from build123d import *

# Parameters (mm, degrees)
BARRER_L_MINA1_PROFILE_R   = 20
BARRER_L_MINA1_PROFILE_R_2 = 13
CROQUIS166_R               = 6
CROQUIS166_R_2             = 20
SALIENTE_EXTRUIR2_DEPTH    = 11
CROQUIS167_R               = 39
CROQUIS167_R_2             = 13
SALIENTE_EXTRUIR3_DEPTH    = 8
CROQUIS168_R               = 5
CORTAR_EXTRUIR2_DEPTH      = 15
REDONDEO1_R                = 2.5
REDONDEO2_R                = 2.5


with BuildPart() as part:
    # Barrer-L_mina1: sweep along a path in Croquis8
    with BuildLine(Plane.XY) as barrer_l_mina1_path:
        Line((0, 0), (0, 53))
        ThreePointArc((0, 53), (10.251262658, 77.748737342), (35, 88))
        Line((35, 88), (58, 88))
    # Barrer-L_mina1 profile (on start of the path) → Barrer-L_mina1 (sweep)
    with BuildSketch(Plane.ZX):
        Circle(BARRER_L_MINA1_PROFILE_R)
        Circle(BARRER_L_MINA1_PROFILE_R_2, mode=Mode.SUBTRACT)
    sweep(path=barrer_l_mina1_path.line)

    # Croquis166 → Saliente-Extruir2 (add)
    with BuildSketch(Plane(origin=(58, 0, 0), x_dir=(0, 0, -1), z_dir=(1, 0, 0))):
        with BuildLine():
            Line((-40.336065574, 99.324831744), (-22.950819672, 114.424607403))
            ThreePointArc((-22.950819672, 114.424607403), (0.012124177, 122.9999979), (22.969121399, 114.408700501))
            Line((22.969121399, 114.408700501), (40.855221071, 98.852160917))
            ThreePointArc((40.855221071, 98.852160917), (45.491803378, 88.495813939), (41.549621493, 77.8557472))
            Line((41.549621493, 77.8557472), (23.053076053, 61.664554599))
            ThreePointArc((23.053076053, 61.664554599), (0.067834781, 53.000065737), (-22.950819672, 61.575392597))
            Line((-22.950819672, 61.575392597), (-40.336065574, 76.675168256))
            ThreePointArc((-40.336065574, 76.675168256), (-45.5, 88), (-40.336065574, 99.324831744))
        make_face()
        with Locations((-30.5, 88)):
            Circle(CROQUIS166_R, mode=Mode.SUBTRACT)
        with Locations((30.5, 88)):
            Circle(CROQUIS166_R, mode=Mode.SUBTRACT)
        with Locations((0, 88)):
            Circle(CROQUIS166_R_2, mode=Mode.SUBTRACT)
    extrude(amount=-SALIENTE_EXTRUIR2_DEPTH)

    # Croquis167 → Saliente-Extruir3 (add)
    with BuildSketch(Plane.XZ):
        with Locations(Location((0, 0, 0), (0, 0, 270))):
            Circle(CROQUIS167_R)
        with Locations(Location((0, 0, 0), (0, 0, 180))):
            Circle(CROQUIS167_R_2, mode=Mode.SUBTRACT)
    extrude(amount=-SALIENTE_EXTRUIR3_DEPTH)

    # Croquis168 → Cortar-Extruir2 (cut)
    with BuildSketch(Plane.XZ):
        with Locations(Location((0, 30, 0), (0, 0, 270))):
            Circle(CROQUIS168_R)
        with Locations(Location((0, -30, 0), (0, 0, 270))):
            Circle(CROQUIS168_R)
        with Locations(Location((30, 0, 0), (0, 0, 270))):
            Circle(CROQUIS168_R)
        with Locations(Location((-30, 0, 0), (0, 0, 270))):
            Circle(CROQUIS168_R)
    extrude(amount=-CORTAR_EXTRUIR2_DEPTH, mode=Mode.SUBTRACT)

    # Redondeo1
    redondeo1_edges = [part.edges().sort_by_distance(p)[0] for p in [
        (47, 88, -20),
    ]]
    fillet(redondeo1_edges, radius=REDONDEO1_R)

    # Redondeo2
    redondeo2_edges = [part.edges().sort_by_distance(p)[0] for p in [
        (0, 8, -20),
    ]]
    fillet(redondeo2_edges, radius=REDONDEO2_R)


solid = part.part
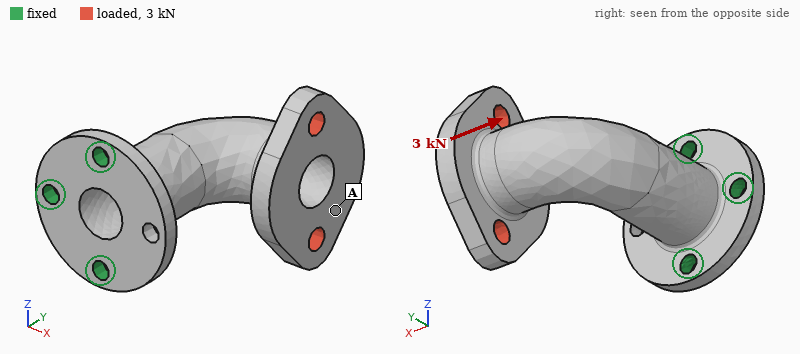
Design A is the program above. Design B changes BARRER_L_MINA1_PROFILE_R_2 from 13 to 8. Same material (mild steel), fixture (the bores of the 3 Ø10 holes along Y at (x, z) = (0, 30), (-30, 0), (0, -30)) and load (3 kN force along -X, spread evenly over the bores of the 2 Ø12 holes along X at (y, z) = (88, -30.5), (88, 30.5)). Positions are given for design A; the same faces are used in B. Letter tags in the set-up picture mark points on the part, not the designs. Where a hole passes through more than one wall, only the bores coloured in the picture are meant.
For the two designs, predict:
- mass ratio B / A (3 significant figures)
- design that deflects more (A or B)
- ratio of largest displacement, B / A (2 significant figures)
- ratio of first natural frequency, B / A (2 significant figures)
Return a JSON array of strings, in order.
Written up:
["1.28", "A", "0.83", "0.99"]
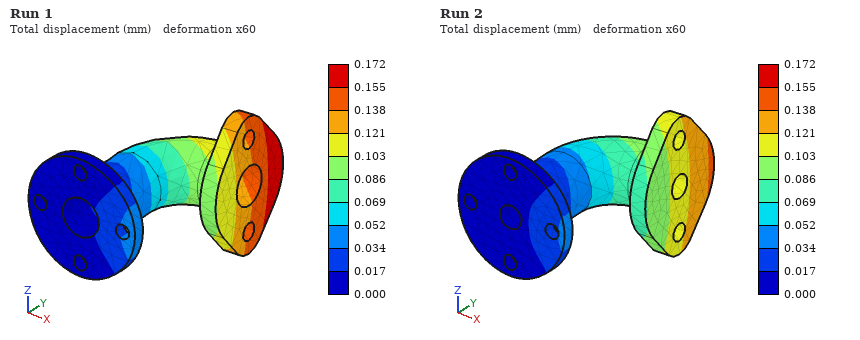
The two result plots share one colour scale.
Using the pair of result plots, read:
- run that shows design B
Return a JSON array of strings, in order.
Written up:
["Run 2"]
